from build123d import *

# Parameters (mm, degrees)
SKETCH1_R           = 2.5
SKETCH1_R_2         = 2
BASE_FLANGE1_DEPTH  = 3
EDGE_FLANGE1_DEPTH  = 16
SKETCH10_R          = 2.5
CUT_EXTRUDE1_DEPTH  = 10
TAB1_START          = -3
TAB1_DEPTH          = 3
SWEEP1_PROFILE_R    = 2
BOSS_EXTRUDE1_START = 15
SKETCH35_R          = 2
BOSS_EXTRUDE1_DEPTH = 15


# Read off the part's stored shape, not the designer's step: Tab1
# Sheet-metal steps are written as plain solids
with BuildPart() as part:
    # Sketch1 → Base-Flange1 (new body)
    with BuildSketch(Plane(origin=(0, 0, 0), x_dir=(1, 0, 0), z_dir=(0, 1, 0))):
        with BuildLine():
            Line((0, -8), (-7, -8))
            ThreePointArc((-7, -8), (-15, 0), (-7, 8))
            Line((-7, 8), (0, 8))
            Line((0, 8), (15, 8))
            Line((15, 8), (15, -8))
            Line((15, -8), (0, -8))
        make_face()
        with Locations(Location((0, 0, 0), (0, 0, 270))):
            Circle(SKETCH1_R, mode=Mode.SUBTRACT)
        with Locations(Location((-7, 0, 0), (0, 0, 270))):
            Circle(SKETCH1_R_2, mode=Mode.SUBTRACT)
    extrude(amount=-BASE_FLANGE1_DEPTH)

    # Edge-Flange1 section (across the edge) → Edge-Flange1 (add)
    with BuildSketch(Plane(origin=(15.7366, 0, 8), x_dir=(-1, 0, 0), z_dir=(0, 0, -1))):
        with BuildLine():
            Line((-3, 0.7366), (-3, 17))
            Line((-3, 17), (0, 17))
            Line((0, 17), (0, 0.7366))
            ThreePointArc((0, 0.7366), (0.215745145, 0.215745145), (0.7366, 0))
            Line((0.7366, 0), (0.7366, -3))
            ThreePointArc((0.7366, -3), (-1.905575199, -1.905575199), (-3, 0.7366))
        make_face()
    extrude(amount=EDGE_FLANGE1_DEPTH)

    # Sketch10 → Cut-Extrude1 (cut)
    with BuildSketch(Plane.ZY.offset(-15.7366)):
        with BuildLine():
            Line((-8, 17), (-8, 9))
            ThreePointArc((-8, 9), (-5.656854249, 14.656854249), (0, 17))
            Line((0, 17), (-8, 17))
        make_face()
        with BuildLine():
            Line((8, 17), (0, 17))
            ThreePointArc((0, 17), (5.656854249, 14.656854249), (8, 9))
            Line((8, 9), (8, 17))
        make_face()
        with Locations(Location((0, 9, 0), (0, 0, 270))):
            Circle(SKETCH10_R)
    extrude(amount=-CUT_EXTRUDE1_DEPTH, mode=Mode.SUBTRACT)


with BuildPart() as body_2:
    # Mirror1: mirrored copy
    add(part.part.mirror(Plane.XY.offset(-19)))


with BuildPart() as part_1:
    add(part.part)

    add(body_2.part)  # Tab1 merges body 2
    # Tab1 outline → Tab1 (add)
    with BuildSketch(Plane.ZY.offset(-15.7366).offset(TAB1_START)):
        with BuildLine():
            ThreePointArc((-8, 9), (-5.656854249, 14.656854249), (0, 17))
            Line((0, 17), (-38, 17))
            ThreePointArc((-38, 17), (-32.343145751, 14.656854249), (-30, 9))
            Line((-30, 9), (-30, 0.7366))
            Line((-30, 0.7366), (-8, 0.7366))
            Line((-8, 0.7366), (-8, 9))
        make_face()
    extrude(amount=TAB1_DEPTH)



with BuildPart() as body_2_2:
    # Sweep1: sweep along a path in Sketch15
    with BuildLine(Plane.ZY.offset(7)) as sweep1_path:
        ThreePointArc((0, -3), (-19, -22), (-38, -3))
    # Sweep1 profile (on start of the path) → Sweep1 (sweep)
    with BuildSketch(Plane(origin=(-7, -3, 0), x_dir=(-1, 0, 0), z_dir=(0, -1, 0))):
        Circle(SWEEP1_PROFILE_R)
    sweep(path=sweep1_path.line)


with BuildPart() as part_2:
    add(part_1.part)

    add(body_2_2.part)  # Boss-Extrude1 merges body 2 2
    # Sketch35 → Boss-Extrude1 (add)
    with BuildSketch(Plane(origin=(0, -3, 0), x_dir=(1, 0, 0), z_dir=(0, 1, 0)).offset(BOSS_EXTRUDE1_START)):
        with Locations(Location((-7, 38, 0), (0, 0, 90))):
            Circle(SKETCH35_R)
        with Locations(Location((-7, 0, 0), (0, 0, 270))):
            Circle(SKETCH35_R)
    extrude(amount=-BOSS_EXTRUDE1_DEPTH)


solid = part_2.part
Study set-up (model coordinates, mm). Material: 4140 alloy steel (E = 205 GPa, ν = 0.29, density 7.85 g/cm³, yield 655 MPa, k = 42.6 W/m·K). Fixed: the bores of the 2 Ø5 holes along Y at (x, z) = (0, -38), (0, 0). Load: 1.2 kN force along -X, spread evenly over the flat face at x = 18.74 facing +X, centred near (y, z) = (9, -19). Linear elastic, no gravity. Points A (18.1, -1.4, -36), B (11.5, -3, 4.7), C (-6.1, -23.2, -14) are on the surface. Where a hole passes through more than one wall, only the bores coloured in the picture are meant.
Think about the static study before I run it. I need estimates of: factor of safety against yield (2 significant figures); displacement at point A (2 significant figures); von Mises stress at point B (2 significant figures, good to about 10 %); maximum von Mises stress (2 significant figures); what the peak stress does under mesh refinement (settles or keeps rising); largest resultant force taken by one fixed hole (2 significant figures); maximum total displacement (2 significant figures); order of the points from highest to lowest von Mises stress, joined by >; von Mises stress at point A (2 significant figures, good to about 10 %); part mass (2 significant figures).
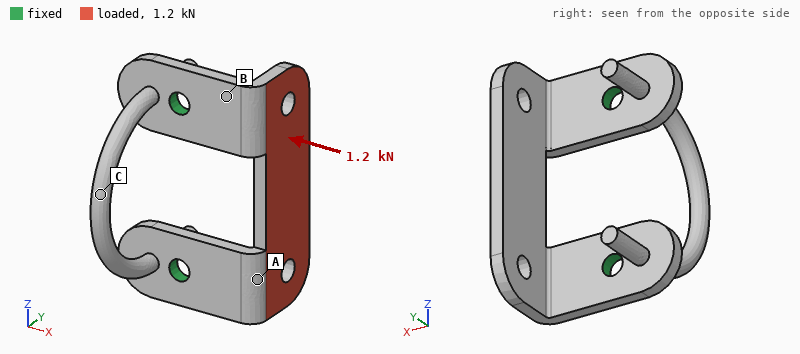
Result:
0.83
0.11 mm
220 MPa
790 MPa
settles
610 N
0.34 mm
B > A > C
150 MPa
50 g
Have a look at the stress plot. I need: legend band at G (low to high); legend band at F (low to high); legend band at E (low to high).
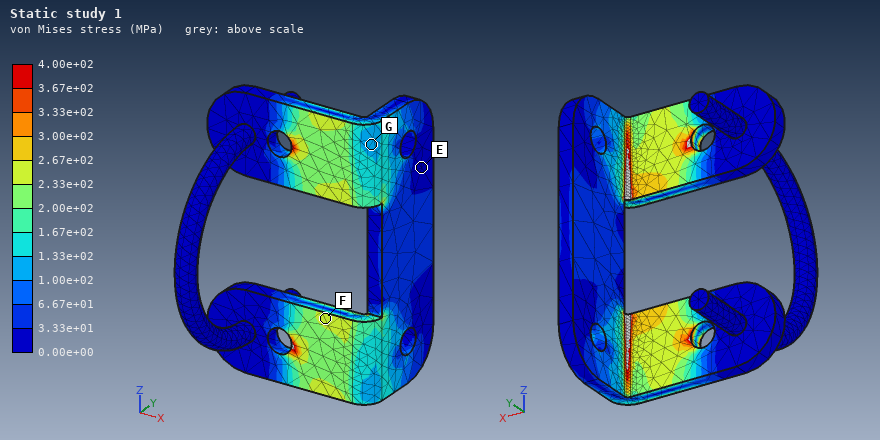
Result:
1.00e+02 to 1.33e+02 MPa
2.33e+02 to 2.67e+02 MPa
0.00e+00 to 3.33e+01 MPa
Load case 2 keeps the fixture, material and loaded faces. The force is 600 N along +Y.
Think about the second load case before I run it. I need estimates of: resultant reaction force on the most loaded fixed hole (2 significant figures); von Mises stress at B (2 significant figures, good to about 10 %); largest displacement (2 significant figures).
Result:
300 N
87 MPa
0.14 mm
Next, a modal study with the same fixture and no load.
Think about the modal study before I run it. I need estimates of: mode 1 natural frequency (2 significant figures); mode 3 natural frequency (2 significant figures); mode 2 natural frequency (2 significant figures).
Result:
2300 Hz
4200 Hz
3300 Hz
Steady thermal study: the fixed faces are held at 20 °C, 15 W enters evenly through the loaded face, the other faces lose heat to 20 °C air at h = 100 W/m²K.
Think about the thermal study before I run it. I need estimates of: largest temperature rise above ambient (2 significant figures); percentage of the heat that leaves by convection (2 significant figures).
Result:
56 K
54 %
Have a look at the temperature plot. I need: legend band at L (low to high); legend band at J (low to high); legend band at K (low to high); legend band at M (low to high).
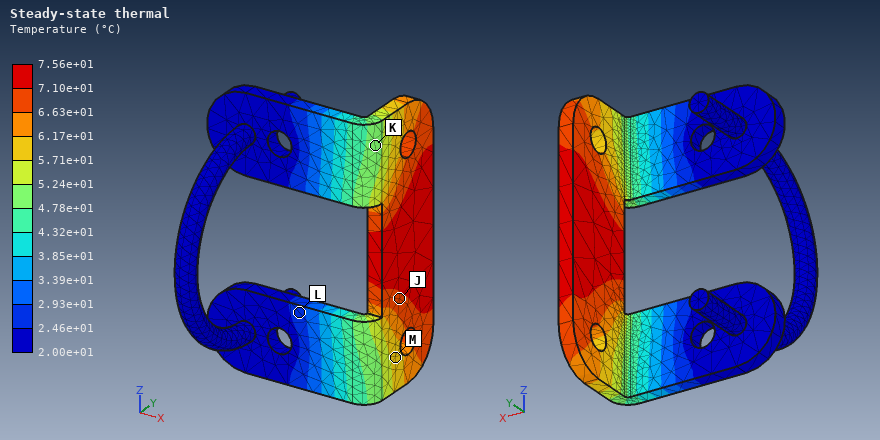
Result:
2.46e+01 to 2.93e+01 °C
6.63e+01 to 7.10e+01 °C
4.78e+01 to 5.24e+01 °C
5.71e+01 to 6.17e+01 °C
